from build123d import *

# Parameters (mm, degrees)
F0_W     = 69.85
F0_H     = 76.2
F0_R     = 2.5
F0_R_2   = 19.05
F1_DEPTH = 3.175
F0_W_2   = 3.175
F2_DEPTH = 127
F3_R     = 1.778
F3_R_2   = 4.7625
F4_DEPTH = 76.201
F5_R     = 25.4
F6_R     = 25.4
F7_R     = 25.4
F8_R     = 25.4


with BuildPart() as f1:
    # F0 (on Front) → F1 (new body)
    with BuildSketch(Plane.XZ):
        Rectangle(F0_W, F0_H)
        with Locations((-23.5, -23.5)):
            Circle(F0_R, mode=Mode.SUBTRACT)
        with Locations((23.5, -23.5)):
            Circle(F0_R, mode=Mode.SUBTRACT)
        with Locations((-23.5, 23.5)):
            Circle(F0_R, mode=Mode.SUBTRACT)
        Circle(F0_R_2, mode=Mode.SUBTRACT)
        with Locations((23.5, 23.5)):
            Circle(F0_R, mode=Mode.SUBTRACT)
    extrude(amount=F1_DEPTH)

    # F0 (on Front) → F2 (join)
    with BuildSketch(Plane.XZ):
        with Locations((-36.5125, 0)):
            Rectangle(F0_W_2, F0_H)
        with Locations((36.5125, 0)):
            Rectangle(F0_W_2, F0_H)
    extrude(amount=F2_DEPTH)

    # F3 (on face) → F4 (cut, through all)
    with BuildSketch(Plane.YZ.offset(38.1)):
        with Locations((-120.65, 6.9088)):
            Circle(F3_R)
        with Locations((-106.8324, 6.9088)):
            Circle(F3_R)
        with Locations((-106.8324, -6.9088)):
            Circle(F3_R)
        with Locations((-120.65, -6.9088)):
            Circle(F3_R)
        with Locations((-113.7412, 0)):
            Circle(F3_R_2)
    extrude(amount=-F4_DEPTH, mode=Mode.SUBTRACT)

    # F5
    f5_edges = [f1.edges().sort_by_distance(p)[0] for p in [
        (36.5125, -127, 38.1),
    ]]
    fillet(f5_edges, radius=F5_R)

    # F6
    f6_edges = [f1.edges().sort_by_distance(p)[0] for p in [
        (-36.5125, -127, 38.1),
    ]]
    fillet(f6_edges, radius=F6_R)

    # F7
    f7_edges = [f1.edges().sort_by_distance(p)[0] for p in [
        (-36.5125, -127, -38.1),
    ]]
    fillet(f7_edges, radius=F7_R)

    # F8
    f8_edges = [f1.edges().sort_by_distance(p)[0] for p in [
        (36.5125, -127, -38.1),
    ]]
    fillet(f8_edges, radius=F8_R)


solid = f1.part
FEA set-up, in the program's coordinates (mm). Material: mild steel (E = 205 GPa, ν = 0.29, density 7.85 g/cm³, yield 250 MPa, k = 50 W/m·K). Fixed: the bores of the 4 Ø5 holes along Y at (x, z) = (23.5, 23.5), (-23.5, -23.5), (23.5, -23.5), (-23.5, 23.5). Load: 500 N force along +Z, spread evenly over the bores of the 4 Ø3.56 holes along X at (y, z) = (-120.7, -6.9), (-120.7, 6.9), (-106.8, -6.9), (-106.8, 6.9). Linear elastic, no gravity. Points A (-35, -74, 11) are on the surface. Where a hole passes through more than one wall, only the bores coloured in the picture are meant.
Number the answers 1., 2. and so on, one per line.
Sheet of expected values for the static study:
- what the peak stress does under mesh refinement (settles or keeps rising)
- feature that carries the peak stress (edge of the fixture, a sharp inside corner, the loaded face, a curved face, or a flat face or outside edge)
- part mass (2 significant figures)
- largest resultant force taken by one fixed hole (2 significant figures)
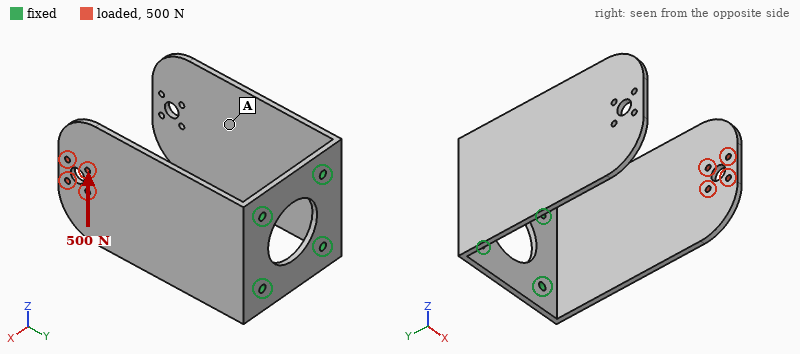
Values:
1. keeps rising
2. edge of the fixture
3. 570 g
4. 1.2 kN
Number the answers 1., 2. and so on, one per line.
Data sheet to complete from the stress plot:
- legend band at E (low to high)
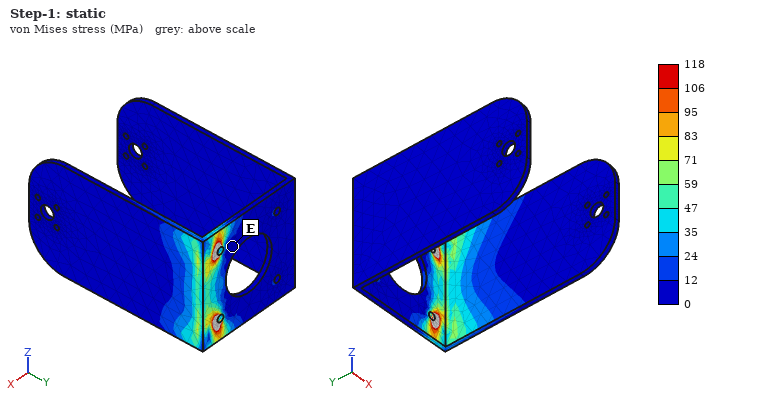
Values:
1. 0 to 12 MPa
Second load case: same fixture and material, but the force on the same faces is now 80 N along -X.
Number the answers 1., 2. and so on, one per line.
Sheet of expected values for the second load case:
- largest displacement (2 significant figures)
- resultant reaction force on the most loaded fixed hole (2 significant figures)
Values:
1. 1.4 mm
2. 60 N
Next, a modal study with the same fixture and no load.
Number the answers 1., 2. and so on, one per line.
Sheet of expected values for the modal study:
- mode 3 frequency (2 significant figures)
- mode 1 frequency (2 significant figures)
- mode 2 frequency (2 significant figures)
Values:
1. 610 Hz
2. 150 Hz
3. 150 Hz
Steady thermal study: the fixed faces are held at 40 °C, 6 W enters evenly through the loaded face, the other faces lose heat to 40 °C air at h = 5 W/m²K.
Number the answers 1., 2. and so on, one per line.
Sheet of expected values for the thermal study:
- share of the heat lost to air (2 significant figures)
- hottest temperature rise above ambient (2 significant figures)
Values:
1. 42 %
2. 52 K
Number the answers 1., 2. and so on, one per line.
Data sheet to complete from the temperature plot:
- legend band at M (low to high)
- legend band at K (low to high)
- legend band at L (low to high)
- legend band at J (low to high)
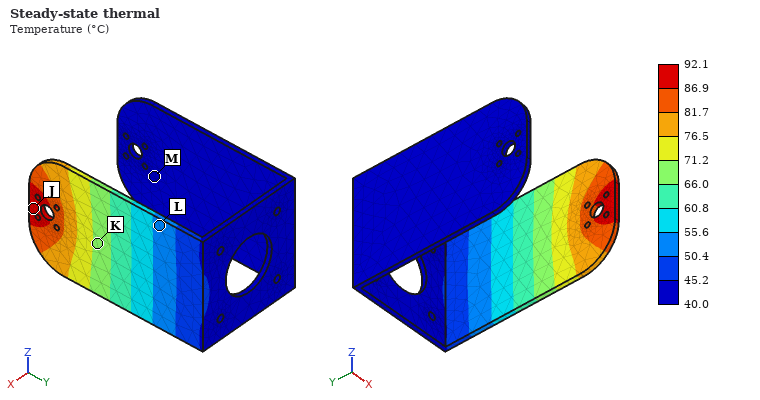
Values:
1. 40.0 to 45.2 °C
2. 66.0 to 71.2 °C
3. 50.4 to 55.6 °C
4. 86.9 to 92.1 °C
